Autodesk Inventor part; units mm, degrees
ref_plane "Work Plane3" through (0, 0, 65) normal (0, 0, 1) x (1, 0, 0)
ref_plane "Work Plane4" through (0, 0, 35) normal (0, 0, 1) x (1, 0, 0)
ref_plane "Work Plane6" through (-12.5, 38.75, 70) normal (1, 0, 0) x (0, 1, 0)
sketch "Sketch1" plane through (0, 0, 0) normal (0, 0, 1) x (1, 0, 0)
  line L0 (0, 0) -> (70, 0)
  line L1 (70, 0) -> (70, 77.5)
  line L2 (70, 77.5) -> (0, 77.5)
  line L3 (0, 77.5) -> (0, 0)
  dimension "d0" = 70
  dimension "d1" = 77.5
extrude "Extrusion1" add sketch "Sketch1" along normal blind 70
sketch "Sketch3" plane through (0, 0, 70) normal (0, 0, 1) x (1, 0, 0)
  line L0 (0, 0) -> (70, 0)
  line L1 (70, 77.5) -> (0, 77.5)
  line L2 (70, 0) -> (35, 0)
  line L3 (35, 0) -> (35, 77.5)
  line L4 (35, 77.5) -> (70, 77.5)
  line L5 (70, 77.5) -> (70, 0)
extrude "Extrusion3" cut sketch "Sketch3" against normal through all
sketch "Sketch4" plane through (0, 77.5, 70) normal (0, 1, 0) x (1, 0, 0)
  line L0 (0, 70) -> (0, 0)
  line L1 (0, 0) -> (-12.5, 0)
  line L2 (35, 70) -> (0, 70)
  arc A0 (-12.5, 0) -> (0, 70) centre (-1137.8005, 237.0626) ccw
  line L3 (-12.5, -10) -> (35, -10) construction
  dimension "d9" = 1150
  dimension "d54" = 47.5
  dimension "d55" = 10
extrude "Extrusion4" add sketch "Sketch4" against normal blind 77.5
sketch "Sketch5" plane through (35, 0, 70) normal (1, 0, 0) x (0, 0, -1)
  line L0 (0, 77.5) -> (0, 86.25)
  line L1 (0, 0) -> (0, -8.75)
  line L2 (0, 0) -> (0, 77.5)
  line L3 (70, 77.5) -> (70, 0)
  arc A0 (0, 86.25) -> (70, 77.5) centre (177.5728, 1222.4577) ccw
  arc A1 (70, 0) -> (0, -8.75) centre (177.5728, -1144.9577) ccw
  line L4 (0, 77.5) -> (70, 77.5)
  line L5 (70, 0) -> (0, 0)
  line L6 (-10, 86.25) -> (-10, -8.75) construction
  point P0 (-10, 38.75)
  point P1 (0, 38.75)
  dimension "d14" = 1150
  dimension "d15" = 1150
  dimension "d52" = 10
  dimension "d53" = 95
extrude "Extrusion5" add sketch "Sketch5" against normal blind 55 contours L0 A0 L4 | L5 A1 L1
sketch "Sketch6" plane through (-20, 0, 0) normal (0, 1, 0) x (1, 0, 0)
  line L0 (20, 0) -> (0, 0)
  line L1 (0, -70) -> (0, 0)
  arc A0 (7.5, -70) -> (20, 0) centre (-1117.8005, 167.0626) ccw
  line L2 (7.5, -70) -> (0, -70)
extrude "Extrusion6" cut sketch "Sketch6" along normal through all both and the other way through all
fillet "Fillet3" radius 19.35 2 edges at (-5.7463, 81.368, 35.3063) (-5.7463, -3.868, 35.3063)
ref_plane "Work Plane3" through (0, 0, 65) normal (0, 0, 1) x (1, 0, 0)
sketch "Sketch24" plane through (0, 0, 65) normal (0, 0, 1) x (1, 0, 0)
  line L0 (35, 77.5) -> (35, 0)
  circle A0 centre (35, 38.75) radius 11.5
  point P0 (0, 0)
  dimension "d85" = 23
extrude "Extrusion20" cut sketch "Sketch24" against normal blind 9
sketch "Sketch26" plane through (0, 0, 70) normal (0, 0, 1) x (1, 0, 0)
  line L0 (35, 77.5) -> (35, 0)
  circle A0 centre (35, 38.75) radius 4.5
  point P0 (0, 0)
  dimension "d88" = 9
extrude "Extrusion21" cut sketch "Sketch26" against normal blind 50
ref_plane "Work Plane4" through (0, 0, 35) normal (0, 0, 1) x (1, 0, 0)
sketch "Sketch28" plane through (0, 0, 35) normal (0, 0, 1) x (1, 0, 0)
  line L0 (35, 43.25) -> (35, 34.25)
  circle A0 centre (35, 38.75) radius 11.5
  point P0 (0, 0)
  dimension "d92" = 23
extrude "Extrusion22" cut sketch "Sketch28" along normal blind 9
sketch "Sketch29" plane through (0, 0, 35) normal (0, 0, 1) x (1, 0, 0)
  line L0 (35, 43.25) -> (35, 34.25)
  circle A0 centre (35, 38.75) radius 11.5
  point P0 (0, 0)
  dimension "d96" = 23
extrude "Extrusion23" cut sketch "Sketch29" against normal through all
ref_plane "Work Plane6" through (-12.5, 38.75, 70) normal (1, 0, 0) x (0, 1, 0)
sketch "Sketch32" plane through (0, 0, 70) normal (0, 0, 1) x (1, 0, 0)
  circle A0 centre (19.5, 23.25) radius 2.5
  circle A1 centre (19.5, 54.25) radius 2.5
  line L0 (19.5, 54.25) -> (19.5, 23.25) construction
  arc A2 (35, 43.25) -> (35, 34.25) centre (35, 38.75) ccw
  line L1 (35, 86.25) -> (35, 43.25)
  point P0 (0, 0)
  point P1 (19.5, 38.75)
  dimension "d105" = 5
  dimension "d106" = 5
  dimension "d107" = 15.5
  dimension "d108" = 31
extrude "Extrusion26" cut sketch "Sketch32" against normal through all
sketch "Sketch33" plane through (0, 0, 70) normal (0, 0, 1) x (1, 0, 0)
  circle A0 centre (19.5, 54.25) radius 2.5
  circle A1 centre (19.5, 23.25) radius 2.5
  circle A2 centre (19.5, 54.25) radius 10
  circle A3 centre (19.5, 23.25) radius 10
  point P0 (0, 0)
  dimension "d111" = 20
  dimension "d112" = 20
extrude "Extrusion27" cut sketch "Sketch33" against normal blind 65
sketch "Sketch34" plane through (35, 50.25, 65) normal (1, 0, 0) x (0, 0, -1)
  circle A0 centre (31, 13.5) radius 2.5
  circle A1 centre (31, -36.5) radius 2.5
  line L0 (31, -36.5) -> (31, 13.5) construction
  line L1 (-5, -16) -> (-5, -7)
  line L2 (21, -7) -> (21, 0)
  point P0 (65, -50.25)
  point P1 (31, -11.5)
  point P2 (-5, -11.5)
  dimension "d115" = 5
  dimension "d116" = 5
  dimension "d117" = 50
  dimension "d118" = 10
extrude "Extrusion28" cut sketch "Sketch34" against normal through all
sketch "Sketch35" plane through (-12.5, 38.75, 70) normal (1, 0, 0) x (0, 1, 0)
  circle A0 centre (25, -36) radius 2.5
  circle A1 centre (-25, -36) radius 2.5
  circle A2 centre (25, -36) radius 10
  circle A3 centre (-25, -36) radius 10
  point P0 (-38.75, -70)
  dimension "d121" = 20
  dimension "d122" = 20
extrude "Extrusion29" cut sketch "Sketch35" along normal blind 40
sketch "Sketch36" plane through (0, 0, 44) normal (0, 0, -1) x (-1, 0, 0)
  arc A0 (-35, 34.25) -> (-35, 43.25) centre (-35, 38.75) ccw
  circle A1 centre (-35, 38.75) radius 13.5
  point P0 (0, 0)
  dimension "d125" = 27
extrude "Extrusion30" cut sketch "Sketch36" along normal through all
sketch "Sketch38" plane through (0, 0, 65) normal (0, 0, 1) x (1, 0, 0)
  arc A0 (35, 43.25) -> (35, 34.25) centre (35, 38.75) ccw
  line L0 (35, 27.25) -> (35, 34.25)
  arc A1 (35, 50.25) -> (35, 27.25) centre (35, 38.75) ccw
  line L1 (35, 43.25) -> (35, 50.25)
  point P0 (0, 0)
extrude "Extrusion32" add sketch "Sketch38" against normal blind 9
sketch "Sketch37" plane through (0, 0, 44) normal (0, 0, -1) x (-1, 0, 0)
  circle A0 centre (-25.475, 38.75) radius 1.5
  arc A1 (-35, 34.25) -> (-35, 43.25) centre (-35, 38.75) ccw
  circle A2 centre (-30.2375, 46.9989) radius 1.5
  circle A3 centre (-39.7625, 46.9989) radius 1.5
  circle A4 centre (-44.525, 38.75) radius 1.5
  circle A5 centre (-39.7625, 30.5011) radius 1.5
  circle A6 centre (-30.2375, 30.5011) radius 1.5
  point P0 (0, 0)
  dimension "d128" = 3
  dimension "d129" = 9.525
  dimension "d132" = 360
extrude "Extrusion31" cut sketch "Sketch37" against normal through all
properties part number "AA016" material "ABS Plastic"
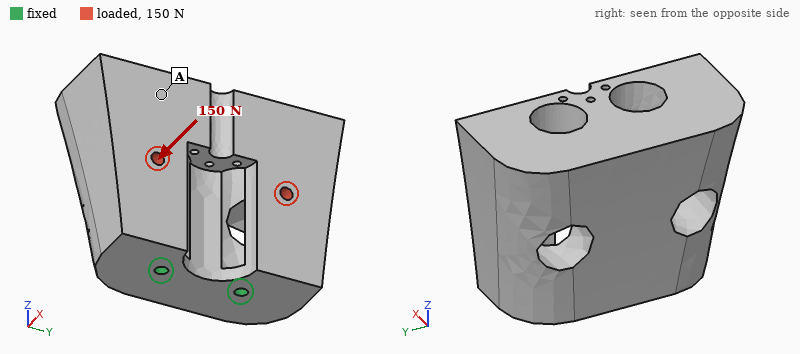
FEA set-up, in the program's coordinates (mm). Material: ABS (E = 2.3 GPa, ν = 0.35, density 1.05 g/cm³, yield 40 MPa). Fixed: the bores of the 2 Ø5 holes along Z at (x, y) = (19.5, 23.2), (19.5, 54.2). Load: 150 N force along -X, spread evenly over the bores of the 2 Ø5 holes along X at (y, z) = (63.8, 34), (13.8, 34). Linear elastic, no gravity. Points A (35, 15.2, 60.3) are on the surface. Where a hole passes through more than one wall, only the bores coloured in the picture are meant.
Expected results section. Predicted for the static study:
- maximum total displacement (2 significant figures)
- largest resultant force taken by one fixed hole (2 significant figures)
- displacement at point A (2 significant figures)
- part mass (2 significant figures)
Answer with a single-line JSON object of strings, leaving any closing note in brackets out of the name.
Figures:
{"maximum total displacement": "0.85 mm", "largest resultant force taken by one fixed hole": "84 N", "displacement at point A": "0.69 mm", "part mass": "170 g"}
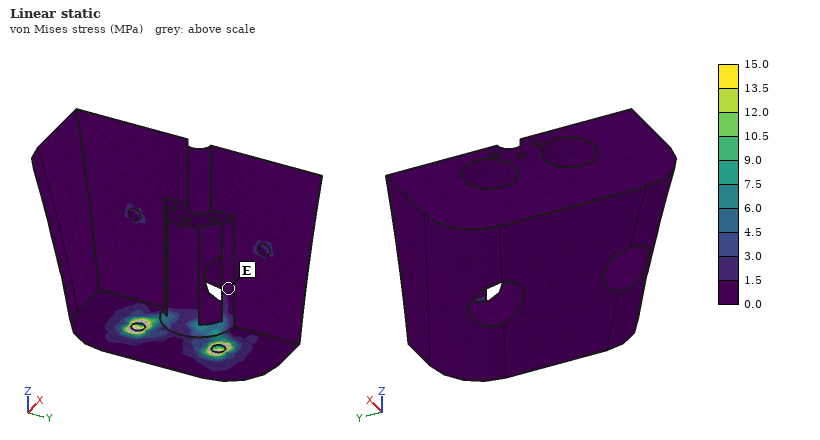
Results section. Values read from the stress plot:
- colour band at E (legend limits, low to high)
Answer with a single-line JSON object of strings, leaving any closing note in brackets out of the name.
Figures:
{"colour band at E": "0.0 to 1.5 MPa"}
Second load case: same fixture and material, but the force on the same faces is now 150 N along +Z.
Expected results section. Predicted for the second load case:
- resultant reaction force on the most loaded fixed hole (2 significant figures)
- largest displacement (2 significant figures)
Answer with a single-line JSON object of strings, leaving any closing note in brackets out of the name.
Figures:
{"resultant reaction force on the most loaded fixed hole": "75 N", "largest displacement": "0.31 mm"}
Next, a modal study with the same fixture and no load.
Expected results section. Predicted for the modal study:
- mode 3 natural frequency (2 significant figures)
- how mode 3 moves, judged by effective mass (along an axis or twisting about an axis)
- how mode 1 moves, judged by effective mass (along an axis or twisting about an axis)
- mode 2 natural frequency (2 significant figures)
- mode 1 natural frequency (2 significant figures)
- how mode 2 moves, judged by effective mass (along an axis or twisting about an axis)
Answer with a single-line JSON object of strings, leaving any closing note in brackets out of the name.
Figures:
{"mode 3 natural frequency": "800 Hz", "how mode 3 moves, judged by effective mass": "twisting about Z", "how mode 1 moves, judged by effective mass": "along X", "mode 2 natural frequency": "410 Hz", "mode 1 natural frequency": "170 Hz", "how mode 2 moves, judged by effective mass": "along Y"}
